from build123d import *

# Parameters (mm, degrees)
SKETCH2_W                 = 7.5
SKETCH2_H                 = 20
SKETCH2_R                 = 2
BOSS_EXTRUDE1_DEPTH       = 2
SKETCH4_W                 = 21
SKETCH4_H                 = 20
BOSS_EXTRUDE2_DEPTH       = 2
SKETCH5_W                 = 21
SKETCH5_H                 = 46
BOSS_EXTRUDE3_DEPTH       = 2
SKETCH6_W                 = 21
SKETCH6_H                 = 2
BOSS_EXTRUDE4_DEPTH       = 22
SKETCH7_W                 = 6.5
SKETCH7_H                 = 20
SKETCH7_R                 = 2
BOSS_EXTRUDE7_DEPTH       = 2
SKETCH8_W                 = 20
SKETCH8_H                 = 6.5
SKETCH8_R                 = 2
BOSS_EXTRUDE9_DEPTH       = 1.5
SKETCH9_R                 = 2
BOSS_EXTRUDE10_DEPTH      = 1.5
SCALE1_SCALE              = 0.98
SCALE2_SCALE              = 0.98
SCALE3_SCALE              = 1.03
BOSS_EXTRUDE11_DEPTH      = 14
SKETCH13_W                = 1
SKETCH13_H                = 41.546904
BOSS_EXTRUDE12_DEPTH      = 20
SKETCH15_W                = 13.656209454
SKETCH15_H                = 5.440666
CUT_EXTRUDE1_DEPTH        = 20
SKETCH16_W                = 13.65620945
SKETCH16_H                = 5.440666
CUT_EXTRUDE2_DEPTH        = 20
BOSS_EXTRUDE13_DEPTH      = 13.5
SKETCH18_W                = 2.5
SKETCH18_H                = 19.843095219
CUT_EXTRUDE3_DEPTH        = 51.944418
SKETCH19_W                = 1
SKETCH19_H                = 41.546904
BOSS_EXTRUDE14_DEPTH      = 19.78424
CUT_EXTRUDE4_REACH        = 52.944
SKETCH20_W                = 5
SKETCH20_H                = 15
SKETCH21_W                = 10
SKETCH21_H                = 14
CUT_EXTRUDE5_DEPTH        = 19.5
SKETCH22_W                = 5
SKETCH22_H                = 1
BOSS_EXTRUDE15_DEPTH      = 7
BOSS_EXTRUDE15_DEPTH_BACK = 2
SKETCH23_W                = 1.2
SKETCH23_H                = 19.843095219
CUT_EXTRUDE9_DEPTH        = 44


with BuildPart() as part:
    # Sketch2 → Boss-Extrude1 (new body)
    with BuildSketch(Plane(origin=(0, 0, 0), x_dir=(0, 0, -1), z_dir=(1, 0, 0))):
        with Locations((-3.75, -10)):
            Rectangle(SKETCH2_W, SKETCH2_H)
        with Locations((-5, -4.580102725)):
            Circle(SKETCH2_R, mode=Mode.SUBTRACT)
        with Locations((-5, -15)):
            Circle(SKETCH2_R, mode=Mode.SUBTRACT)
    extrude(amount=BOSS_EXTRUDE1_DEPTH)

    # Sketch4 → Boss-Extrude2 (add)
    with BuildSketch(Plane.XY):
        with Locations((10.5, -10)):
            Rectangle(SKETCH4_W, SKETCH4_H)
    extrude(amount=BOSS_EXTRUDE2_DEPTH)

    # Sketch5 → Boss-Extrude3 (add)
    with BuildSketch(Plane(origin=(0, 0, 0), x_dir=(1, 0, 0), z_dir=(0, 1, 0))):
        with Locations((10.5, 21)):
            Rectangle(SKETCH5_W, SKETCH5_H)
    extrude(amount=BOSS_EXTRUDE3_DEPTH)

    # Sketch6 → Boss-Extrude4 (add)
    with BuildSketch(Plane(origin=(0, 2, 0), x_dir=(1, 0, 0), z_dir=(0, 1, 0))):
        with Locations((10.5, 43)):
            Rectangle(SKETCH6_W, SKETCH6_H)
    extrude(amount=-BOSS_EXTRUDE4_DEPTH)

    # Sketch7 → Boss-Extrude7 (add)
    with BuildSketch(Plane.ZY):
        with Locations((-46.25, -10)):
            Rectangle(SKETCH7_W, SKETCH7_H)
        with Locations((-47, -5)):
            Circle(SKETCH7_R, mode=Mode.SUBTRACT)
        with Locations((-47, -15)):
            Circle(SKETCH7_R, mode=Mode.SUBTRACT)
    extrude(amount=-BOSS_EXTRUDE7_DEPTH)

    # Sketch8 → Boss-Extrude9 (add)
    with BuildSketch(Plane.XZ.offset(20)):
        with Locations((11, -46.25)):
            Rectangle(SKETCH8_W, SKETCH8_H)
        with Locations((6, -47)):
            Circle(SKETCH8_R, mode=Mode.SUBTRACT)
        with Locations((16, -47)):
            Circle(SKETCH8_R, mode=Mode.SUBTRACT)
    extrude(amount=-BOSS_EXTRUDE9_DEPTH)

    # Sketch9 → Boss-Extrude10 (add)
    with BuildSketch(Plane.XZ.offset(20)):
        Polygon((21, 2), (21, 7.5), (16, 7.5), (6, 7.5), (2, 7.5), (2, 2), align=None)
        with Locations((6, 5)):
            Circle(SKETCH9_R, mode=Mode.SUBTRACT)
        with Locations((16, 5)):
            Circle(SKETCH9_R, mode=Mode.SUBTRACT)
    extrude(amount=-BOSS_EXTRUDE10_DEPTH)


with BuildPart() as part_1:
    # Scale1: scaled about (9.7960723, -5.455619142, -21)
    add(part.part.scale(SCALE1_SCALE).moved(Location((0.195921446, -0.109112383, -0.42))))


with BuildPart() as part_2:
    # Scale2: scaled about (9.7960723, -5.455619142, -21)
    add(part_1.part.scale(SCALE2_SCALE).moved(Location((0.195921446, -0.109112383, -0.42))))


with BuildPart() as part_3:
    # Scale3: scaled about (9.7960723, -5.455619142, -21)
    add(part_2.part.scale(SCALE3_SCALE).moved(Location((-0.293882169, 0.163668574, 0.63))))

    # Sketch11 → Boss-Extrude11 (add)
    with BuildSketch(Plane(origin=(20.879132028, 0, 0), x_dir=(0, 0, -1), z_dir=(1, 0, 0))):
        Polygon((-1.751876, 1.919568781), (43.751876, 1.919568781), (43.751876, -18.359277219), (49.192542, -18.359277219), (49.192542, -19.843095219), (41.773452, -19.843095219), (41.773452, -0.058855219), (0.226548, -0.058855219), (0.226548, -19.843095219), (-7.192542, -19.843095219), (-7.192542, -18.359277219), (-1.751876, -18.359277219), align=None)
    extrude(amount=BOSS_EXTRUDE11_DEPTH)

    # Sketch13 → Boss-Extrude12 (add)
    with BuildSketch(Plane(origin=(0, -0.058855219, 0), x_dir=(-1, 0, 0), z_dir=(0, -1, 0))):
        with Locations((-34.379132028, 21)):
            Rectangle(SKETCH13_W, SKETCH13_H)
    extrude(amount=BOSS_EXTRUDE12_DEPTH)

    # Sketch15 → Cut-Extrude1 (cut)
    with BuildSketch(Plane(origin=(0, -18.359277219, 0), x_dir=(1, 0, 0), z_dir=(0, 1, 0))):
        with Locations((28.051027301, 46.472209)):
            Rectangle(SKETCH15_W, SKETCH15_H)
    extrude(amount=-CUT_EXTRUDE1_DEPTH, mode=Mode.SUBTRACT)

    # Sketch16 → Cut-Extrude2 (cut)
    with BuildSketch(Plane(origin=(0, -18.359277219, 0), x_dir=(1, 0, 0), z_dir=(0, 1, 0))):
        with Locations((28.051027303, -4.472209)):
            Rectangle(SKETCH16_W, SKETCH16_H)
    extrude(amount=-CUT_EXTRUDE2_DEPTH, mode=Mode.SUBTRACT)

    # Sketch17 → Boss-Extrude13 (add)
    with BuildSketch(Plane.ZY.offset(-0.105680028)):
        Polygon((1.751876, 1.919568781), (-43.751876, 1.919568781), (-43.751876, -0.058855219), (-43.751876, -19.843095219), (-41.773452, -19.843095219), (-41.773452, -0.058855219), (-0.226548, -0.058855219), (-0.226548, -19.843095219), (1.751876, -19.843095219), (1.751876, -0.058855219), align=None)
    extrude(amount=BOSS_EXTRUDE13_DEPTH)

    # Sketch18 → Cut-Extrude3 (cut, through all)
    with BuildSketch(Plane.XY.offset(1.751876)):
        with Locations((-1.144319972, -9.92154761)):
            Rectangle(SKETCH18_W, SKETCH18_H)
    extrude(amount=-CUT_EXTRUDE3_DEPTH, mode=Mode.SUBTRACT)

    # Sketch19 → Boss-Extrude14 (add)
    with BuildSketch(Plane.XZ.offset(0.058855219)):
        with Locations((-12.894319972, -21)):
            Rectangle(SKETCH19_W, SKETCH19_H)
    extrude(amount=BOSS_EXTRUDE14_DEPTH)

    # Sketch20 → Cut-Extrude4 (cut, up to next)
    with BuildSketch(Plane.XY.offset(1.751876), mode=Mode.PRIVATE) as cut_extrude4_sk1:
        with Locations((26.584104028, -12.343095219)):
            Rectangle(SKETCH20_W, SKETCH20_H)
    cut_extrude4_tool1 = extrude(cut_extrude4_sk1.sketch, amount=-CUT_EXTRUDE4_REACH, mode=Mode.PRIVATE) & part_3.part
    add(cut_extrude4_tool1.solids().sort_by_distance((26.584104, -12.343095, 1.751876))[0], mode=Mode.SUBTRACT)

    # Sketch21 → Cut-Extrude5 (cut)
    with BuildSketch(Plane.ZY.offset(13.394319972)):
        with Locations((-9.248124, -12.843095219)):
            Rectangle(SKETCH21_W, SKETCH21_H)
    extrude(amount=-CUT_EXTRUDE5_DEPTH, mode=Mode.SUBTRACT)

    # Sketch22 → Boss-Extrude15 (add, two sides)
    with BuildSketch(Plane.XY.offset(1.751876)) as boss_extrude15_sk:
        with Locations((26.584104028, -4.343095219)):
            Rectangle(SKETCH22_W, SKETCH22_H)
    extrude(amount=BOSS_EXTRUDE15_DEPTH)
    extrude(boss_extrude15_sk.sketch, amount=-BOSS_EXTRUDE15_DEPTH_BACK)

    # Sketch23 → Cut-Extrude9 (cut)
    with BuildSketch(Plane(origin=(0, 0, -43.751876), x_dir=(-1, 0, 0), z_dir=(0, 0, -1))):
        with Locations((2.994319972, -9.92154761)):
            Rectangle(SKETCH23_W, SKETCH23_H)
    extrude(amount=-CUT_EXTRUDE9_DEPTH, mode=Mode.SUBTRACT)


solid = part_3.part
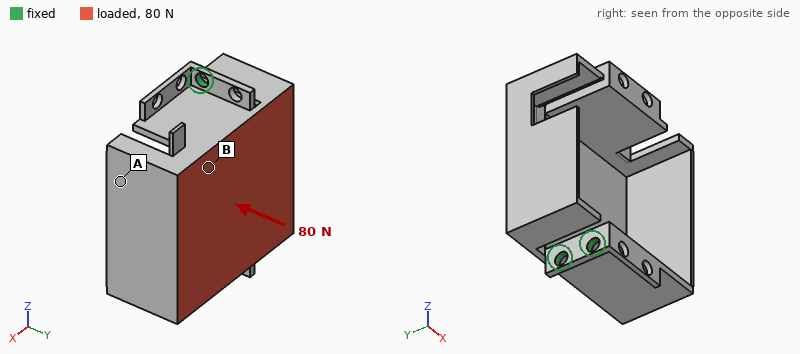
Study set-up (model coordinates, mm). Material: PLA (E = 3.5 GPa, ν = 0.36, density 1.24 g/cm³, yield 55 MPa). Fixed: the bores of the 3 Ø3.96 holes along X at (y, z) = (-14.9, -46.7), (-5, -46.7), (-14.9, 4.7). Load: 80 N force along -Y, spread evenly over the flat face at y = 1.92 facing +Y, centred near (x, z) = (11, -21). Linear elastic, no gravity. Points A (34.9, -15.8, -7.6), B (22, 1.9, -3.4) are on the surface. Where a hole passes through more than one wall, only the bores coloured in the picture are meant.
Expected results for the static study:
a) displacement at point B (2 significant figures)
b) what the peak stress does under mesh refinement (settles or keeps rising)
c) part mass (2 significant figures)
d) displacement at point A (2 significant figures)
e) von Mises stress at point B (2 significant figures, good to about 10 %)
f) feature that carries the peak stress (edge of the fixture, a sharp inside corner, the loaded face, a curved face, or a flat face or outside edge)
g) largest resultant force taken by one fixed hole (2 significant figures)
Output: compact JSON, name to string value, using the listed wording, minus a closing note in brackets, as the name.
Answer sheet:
{"displacement at point B": "0.28 mm", "what the peak stress does under mesh refinement": "keeps rising", "part mass": "12 g", "displacement at point A": "0.36 mm", "von Mises stress at point B": "2.7 MPa", "feature that carries the peak stress": "a sharp inside corner", "largest resultant force taken by one fixed hole": "44 N"}
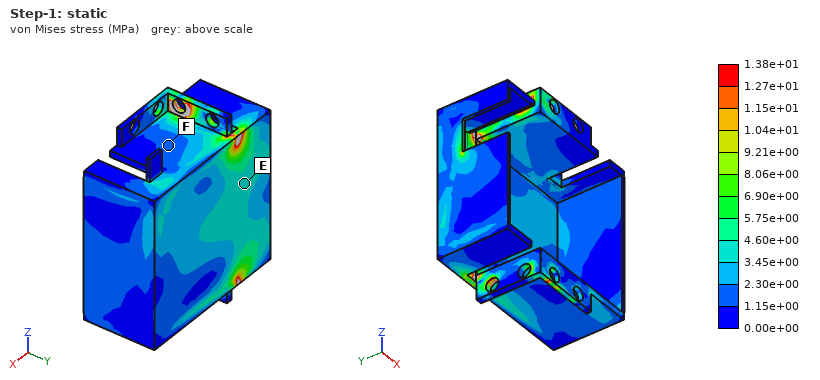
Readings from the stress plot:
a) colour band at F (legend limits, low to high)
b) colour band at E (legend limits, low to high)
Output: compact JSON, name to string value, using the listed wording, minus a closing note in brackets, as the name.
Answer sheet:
{"colour band at F": "1.15e+00 to 2.30e+00 MPa", "colour band at E": "3.45e+00 to 4.60e+00 MPa"}
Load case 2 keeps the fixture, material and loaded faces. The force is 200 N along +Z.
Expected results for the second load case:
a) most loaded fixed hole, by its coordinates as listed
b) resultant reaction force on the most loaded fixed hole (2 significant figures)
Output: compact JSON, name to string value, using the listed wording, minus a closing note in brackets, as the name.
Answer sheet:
{"most loaded fixed hole, by its coordinates as listed": "(-5, -46.7)", "resultant reaction force on the most loaded fixed hole": "190 N"}
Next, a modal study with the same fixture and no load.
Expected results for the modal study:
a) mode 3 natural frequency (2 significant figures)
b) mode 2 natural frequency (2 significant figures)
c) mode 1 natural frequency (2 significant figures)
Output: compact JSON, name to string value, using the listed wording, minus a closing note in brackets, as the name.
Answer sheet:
{"mode 3 natural frequency": "760 Hz", "mode 2 natural frequency": "580 Hz", "mode 1 natural frequency": "530 Hz"}
